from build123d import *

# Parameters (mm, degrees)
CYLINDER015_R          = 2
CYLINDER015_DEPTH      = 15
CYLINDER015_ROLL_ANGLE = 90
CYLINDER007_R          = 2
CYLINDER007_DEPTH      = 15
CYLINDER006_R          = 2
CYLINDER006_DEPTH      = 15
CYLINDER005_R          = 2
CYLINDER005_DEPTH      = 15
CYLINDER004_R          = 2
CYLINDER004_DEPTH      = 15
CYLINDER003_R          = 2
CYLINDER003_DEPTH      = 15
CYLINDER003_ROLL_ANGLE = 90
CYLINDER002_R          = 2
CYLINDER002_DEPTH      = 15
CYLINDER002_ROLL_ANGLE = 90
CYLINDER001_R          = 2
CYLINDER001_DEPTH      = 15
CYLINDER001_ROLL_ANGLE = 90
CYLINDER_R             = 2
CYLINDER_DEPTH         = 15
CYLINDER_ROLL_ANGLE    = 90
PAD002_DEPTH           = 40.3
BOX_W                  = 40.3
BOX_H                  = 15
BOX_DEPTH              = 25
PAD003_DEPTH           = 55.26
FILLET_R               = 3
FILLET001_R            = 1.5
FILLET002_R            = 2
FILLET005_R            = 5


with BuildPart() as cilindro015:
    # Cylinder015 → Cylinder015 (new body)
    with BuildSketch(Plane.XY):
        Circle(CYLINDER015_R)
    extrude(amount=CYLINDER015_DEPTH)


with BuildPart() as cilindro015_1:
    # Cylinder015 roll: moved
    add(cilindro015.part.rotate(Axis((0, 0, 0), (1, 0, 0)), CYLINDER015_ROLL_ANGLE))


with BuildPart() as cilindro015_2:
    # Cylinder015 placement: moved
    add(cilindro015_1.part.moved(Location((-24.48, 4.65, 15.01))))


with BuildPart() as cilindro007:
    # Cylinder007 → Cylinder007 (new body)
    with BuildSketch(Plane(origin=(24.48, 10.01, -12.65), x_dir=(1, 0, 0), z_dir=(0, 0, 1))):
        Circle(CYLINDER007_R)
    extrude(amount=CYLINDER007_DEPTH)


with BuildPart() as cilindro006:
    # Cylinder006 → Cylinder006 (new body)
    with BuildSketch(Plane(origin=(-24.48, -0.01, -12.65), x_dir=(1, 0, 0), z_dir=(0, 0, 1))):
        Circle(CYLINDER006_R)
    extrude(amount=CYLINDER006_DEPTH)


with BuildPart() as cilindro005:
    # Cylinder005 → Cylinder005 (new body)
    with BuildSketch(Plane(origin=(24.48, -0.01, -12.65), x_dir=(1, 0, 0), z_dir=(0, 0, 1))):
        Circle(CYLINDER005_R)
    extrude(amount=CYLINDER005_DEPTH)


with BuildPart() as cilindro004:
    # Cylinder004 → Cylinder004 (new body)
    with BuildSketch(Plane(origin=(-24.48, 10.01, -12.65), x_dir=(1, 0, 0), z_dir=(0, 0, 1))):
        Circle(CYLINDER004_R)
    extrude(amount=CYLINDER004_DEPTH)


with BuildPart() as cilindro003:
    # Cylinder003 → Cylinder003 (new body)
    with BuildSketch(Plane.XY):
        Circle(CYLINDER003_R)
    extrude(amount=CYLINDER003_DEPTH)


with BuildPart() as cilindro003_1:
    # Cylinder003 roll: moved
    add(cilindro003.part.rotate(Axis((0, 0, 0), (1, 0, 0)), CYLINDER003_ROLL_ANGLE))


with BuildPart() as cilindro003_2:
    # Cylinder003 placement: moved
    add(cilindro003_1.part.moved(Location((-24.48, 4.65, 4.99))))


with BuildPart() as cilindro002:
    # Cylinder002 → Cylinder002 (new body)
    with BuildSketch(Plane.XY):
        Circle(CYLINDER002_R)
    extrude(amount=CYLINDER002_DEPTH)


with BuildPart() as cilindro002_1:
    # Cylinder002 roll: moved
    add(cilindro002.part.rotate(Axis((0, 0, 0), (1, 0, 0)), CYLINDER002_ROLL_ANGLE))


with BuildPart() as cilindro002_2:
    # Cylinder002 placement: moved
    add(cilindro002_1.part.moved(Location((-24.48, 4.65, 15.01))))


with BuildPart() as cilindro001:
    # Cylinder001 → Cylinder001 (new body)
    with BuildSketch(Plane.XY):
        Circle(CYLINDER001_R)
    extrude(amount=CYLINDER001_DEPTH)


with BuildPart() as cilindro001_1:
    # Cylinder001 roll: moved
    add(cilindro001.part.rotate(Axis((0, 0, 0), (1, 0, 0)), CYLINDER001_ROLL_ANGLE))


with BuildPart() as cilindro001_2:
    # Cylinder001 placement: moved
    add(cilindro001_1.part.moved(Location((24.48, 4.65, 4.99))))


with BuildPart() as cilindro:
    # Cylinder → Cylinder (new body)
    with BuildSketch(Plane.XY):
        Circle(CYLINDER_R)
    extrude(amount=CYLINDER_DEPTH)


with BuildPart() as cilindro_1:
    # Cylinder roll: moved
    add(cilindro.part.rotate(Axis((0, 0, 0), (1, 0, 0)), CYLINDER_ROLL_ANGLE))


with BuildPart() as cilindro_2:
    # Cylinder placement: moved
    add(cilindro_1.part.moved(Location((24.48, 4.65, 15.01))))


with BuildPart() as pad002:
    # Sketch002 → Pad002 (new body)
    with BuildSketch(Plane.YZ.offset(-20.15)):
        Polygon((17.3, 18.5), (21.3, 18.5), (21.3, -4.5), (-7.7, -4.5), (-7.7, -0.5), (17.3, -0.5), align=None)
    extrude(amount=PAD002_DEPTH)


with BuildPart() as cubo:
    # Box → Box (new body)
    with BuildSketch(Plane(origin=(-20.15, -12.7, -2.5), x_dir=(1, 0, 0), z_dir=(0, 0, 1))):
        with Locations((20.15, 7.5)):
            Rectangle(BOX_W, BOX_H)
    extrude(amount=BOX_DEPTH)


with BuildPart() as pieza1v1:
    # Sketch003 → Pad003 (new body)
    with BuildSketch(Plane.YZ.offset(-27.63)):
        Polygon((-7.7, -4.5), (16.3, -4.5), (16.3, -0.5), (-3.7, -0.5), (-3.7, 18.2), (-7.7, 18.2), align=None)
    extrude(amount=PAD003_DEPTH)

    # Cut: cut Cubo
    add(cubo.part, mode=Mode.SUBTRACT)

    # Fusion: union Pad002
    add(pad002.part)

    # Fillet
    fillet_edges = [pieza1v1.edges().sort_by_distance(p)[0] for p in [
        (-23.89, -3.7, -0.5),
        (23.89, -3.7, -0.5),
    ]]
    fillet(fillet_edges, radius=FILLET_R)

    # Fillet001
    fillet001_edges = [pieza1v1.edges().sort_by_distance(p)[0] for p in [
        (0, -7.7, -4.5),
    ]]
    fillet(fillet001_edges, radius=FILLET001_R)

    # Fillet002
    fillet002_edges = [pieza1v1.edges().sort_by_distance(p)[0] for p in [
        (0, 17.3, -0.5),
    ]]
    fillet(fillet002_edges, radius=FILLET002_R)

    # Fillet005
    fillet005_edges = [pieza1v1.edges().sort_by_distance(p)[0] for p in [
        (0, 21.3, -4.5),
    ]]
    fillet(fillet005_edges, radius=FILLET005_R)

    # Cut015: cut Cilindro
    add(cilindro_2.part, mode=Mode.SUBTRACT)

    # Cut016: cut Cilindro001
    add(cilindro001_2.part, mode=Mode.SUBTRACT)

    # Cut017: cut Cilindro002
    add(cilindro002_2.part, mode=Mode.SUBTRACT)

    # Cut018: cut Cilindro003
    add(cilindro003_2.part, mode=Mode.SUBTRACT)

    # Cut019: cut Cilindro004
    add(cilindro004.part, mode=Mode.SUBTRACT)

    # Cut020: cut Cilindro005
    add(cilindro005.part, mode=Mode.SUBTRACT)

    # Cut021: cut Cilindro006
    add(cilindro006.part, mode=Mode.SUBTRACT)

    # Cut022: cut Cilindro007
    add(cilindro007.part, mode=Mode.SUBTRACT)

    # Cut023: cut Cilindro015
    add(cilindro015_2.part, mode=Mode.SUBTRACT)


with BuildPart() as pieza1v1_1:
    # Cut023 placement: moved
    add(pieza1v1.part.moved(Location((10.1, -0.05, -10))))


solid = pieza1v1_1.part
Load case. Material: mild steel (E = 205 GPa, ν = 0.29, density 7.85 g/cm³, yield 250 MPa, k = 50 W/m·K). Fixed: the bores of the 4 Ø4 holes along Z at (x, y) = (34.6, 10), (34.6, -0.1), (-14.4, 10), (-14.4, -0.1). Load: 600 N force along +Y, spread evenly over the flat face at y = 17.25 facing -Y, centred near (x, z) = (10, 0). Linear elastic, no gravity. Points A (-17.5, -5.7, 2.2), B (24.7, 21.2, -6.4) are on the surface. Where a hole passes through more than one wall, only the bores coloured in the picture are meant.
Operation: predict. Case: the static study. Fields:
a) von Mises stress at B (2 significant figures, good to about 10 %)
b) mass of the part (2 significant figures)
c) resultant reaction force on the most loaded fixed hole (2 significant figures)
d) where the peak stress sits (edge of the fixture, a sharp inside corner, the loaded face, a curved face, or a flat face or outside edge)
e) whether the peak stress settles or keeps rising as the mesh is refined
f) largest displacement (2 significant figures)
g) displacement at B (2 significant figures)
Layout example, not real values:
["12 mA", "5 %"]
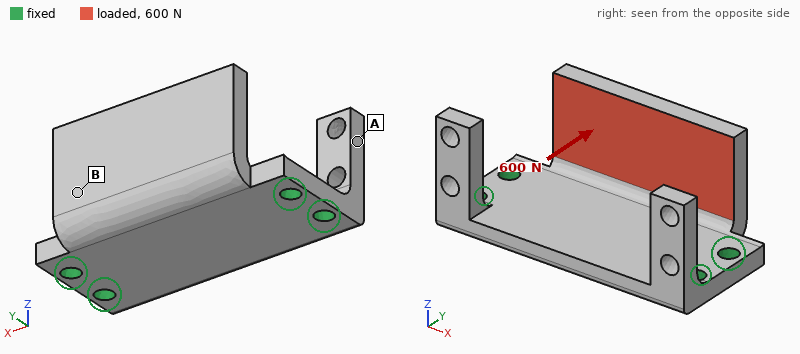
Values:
["34 MPa", "76 g", "280 N", "edge of the fixture", "keeps rising", "55 µm", "20 µm"]
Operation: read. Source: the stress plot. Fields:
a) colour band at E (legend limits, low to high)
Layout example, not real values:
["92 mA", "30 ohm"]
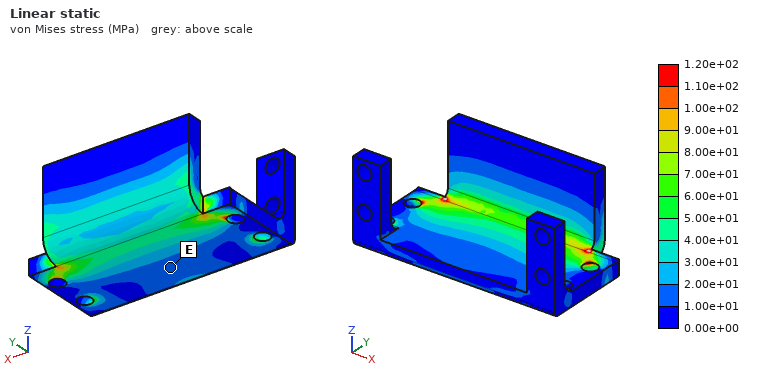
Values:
["1.00e+01 to 2.00e+01 MPa"]
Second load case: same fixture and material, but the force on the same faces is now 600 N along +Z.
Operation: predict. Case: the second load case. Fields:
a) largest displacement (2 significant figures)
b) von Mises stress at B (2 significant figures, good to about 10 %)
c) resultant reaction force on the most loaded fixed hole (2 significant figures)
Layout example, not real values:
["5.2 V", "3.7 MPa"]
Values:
["13 µm", "8.4 MPa", "380 N"]
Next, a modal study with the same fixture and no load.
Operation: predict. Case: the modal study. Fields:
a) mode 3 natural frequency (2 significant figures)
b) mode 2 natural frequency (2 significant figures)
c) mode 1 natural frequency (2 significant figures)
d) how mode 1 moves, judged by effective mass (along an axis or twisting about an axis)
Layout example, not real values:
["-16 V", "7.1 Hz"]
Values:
["7500 Hz", "7500 Hz", "4100 Hz", "along Y"]
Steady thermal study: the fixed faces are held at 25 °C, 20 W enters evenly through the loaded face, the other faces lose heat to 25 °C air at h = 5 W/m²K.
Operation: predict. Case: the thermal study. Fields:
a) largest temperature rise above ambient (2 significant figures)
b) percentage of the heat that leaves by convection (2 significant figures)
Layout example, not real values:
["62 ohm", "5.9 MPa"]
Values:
["67 K", "3.0 %"]
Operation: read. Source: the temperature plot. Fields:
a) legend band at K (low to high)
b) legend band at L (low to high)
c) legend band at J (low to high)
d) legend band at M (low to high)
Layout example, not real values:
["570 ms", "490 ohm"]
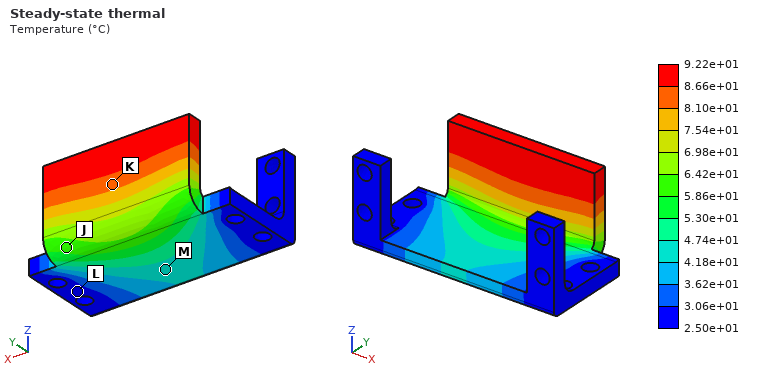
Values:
["8.10e+01 to 8.66e+01 °C", "2.50e+01 to 3.06e+01 °C", "5.86e+01 to 6.42e+01 °C", "4.18e+01 to 4.74e+01 °C"]
